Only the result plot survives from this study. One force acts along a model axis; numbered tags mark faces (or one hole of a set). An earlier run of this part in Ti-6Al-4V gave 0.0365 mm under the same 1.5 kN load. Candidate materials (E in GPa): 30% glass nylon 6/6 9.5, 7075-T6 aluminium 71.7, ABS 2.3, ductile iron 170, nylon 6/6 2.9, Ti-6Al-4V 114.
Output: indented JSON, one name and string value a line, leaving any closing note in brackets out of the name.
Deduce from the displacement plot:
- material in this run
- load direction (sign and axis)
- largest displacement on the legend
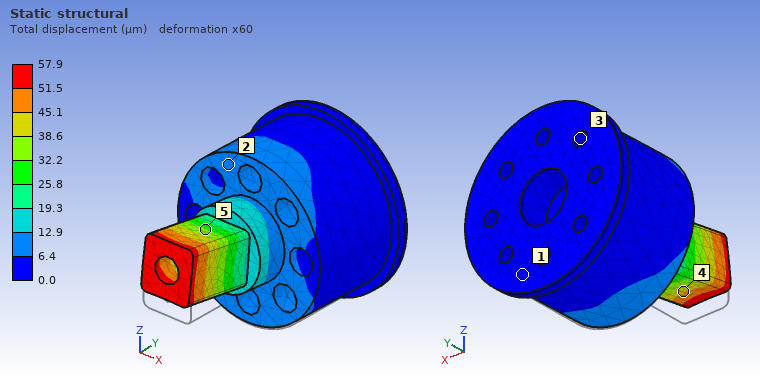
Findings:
{
  "material in this run": "7075-T6 aluminium",
  "load direction": "+Z",
  "largest displacement on the legend": "57.9 µm"
}
